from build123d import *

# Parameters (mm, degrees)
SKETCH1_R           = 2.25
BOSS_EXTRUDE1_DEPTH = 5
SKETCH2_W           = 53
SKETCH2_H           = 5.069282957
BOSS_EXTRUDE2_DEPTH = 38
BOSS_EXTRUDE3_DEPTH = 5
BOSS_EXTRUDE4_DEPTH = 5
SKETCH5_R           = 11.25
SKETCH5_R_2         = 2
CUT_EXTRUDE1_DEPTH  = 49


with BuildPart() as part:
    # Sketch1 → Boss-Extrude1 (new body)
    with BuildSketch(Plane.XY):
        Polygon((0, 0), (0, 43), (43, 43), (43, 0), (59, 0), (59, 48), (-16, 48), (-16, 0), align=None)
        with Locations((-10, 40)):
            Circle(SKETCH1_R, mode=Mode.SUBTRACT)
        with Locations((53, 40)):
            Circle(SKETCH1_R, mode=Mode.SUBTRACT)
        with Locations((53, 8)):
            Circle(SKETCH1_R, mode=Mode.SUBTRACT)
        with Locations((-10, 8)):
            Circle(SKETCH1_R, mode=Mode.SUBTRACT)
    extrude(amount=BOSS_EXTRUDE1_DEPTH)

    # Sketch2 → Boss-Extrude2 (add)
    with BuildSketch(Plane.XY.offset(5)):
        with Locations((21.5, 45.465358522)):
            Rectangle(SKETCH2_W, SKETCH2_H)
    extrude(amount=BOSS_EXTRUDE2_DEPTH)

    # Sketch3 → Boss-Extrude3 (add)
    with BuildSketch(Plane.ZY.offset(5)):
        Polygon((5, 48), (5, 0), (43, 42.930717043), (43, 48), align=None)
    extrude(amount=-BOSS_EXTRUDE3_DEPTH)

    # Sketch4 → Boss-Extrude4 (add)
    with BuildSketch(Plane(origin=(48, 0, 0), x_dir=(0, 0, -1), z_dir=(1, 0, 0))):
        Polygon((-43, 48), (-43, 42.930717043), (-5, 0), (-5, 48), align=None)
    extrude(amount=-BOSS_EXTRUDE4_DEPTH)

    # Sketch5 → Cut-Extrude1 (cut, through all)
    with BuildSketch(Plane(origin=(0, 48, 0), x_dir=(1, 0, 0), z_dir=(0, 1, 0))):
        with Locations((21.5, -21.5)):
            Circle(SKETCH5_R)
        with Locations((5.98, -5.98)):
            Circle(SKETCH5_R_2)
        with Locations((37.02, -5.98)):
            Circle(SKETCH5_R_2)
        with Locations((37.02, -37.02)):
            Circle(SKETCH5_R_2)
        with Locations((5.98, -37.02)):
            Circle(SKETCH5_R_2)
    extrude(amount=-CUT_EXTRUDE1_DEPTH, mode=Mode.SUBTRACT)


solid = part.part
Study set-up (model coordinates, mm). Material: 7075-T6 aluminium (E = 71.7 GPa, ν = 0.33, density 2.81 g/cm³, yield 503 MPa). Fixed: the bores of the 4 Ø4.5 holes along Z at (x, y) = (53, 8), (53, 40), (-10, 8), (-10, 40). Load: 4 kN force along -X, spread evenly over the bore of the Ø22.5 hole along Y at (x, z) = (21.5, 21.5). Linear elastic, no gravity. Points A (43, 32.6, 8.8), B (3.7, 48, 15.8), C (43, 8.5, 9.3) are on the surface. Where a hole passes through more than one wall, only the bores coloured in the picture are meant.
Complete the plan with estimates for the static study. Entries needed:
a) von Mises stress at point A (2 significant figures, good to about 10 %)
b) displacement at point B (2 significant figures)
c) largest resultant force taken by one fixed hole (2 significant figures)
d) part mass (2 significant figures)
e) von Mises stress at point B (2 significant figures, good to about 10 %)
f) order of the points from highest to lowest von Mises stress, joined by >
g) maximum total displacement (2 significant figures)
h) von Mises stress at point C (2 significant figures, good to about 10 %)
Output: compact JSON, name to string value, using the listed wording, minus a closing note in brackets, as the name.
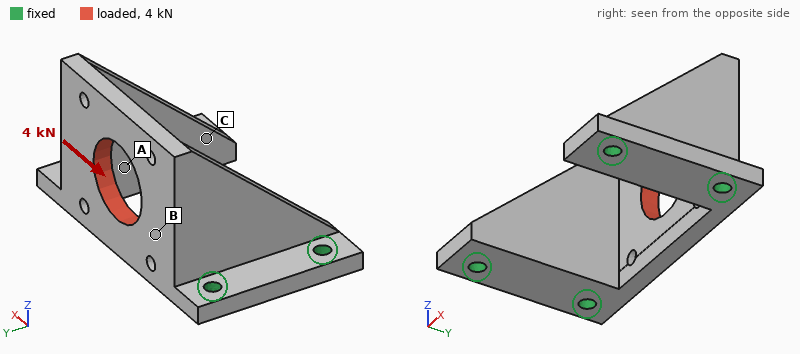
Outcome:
{"von Mises stress at point A": "21 MPa", "displacement at point B": "26 µm", "largest resultant force taken by one fixed hole": "2.5 kN", "part mass": "69 g", "von Mises stress at point B": "33 MPa", "order of the points from highest to lowest von Mises stress, joined by >": "B > A > C", "maximum total displacement": "54 µm", "von Mises stress at point C": "7.9 MPa"}
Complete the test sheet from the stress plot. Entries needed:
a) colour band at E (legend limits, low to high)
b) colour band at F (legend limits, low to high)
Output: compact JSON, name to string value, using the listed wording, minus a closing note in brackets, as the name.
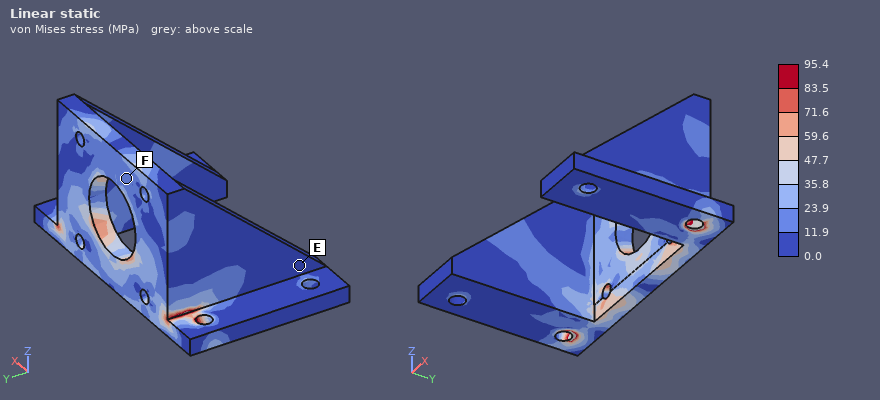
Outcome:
{"colour band at E": "0.0 to 11.9 MPa", "colour band at F": "11.9 to 23.9 MPa"}
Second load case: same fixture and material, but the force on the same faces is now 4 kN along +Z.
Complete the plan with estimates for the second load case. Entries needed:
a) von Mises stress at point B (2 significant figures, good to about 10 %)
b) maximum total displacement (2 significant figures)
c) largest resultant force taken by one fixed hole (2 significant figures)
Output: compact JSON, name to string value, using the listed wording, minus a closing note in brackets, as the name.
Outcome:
{"von Mises stress at point B": "27 MPa", "maximum total displacement": "55 µm", "largest resultant force taken by one fixed hole": "2.4 kN"}
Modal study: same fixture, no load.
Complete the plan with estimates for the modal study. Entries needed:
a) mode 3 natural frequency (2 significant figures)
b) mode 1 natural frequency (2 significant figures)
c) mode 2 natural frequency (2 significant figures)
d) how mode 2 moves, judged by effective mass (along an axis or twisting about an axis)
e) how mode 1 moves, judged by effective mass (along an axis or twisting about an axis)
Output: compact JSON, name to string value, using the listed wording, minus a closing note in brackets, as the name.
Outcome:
{"mode 3 natural frequency": "9200 Hz", "mode 1 natural frequency": "6000 Hz", "mode 2 natural frequency": "7400 Hz", "how mode 2 moves, judged by effective mass": "along X", "how mode 1 moves, judged by effective mass": "along Y"}
